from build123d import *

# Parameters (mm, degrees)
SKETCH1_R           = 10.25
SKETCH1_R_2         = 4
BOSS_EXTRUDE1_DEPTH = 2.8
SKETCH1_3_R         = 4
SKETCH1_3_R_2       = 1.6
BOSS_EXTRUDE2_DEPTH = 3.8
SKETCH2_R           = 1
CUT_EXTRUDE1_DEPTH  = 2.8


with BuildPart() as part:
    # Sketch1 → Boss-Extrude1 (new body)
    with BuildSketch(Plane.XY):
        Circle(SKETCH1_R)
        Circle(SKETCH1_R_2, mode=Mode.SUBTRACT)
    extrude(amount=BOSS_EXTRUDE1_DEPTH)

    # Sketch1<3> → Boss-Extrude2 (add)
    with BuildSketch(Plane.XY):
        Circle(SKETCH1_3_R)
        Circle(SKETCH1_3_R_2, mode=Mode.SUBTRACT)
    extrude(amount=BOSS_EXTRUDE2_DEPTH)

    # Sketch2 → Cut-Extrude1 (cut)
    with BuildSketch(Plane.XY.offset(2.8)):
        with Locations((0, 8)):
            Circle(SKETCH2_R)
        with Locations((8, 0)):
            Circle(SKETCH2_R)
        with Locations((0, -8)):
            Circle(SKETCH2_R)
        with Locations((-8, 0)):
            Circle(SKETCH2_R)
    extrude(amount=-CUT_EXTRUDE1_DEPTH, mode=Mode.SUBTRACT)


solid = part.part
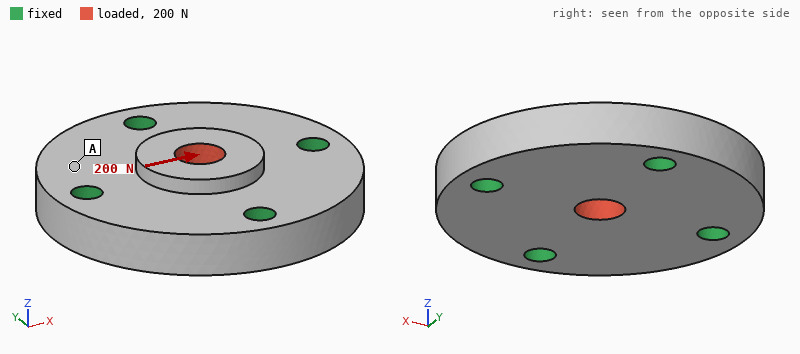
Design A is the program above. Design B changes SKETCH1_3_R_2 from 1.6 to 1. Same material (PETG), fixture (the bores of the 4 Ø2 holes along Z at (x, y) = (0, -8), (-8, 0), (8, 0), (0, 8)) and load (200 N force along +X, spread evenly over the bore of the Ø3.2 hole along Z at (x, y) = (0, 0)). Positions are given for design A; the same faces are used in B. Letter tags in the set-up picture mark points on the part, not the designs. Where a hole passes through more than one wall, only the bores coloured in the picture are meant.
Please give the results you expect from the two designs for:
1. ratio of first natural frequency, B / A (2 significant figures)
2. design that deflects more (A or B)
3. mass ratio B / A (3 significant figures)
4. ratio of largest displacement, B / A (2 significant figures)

0.99
B
1.02
1.1
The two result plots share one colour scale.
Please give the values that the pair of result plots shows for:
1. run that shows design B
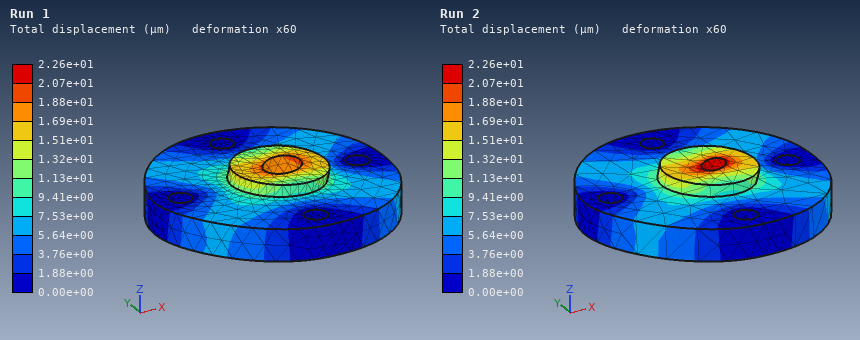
Run 2
